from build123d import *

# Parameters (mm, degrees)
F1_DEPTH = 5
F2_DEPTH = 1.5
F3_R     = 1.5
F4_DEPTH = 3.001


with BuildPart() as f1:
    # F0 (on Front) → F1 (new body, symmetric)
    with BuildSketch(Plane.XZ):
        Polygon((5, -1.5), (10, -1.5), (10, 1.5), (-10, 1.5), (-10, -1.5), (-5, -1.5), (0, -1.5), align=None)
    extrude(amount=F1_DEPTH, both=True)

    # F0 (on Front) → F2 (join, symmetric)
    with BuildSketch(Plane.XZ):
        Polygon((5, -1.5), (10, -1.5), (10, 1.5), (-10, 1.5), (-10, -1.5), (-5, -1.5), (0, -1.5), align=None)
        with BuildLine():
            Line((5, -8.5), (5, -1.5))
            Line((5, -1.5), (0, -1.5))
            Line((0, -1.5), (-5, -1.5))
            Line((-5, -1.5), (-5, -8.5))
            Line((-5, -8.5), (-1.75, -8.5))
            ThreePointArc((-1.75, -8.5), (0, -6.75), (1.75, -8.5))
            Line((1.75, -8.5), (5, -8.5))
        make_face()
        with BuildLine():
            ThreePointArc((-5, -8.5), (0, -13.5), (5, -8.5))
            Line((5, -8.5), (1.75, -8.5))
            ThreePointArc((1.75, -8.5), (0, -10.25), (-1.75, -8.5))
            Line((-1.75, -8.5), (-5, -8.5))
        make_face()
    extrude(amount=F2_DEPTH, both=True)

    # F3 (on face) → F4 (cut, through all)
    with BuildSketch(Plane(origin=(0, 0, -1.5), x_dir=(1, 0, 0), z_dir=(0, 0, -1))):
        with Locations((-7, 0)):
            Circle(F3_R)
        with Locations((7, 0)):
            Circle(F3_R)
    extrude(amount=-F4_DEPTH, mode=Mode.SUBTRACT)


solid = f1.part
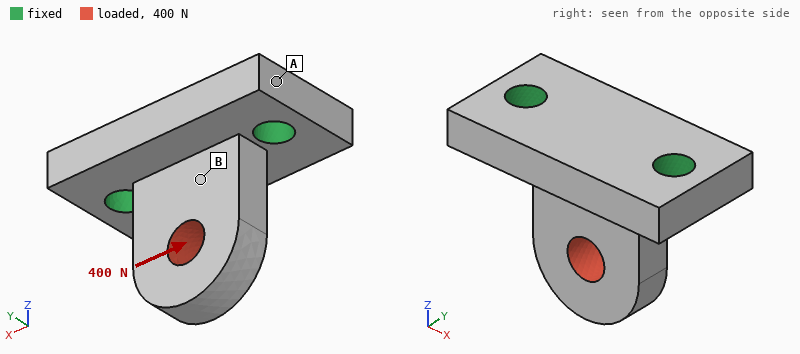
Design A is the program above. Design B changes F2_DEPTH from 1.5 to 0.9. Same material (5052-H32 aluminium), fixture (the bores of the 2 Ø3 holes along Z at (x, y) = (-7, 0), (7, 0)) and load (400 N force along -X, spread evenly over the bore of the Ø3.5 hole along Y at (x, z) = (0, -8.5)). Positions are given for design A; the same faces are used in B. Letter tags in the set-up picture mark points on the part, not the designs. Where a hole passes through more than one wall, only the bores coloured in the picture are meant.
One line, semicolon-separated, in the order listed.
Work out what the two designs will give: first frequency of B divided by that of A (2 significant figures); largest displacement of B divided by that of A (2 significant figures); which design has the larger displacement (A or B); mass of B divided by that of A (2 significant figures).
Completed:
0.73; 1.5; B; 0.86
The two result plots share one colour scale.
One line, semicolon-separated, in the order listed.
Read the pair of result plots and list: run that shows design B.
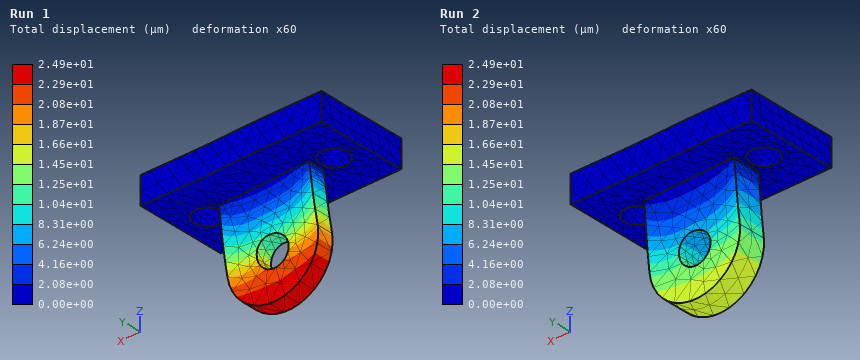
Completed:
Run 1
